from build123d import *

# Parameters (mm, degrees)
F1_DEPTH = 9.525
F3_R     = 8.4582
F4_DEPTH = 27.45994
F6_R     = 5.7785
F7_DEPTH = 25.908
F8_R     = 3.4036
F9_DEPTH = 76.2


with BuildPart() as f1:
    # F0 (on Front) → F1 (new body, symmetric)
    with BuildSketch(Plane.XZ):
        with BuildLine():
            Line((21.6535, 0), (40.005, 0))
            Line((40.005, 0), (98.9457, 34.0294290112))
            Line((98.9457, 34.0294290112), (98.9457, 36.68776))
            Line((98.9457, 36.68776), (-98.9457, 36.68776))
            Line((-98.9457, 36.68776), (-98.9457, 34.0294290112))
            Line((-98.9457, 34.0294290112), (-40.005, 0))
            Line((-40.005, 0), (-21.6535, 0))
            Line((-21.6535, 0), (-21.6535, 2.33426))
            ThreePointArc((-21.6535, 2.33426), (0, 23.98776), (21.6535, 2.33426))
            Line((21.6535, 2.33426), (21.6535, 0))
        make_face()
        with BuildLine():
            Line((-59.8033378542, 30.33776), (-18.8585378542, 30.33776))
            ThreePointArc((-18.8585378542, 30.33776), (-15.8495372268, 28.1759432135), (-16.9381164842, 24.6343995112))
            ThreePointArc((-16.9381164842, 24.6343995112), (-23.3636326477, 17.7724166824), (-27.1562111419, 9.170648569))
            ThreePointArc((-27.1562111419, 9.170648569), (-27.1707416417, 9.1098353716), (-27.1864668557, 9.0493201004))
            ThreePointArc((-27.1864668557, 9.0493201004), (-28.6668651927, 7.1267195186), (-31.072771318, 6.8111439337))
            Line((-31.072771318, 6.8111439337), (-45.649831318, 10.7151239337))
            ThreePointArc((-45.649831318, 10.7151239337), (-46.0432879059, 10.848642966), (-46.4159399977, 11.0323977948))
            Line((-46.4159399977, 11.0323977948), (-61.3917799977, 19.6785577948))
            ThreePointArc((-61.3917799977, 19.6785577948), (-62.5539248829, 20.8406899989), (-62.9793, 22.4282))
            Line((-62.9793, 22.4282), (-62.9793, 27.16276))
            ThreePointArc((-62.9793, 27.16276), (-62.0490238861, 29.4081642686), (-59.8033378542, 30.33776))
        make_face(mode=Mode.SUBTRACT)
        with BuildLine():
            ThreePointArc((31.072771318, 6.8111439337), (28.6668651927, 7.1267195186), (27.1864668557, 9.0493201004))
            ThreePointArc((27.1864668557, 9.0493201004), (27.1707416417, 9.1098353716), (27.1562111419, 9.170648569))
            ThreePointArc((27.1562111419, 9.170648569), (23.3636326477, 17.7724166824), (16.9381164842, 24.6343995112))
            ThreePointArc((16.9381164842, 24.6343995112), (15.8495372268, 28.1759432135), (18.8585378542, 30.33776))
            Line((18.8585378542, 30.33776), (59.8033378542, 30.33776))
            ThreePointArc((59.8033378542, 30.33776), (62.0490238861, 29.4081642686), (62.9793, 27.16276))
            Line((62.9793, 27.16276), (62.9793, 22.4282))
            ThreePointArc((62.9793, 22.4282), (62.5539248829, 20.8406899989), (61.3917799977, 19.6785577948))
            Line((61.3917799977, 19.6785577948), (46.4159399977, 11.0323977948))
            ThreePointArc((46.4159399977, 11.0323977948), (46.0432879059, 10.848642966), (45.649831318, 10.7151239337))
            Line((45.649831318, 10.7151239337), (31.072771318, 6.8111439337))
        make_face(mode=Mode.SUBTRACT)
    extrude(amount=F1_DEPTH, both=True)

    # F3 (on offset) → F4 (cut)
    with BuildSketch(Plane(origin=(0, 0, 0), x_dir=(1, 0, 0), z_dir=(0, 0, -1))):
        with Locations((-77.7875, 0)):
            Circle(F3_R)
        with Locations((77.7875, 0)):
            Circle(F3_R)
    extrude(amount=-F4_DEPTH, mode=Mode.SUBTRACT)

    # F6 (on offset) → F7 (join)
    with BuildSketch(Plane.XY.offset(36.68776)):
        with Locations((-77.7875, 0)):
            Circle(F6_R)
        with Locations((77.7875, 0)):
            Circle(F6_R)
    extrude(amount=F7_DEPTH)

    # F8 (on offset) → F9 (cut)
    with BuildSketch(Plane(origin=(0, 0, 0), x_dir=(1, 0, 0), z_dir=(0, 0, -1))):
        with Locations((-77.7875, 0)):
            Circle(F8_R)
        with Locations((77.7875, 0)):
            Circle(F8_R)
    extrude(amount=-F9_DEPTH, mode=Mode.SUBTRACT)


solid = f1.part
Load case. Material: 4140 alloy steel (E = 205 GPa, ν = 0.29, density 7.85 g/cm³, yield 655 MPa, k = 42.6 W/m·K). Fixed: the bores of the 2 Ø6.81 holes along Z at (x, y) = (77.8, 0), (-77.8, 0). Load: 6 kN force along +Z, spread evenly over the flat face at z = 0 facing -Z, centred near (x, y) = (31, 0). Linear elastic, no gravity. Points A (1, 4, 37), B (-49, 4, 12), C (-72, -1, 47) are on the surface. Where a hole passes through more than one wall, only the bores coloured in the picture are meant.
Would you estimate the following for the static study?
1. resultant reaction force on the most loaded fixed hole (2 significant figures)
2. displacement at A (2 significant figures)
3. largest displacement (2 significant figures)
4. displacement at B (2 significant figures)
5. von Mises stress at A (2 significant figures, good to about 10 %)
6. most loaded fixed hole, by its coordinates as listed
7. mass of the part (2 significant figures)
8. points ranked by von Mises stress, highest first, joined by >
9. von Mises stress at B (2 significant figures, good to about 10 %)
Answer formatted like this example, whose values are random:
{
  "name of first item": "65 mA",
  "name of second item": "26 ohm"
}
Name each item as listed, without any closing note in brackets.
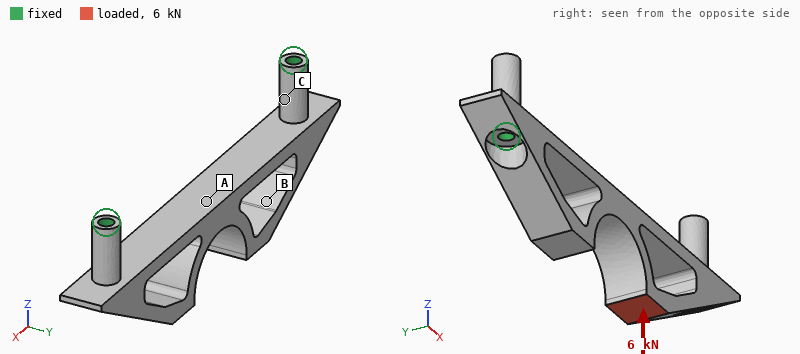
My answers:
{
  "resultant reaction force on the most loaded fixed hole": "4.5 kN",
  "displacement at A": "0.26 mm",
  "largest displacement": "0.27 mm",
  "displacement at B": "0.085 mm",
  "von Mises stress at A": "120 MPa",
  "most loaded fixed hole, by its coordinates as listed": "(77.8, 0)",
  "mass of the part": "430 g",
  "points ranked by von Mises stress, highest first, joined by >": "A > B > C",
  "von Mises stress at B": "64 MPa"
}
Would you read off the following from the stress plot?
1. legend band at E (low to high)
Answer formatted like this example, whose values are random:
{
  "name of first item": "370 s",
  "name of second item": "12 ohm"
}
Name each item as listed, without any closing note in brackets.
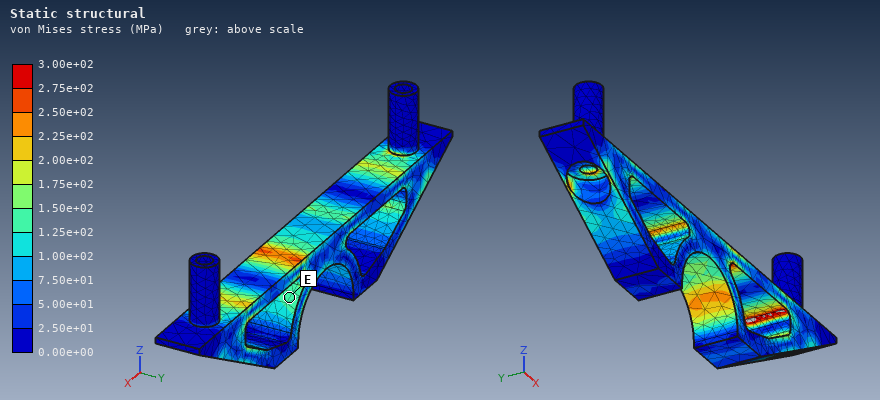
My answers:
{
  "legend band at E": "1.25e+02 to 1.50e+02 MPa"
}
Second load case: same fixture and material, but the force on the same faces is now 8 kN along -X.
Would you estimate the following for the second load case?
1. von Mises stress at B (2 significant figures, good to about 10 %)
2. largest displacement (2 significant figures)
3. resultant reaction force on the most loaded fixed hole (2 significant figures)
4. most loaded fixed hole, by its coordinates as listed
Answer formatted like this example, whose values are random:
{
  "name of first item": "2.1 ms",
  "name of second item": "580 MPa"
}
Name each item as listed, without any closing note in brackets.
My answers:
{
  "von Mises stress at B": "57 MPa",
  "largest displacement": "0.21 mm",
  "resultant reaction force on the most loaded fixed hole": "6.2 kN",
  "most loaded fixed hole, by its coordinates as listed": "(77.8, 0)"
}
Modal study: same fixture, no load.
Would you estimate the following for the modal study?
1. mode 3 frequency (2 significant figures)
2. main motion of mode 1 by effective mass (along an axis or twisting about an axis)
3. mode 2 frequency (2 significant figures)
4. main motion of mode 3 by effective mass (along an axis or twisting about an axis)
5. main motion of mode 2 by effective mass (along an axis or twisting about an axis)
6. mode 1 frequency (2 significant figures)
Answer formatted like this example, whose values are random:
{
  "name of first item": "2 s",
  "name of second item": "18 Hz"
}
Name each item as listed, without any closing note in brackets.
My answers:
{
  "mode 3 frequency": "4500 Hz",
  "main motion of mode 1 by effective mass": "along Z",
  "mode 2 frequency": "2600 Hz",
  "main motion of mode 3 by effective mass": "twisting about X",
  "main motion of mode 2 by effective mass": "along Y",
  "mode 1 frequency": "1600 Hz"
}
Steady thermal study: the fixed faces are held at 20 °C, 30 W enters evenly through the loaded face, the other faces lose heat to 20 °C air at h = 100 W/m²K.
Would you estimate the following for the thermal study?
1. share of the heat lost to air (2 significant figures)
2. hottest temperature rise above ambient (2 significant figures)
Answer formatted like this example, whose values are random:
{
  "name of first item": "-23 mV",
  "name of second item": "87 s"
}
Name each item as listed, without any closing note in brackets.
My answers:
{
  "share of the heat lost to air": "78 %",
  "hottest temperature rise above ambient": "80 K"
}
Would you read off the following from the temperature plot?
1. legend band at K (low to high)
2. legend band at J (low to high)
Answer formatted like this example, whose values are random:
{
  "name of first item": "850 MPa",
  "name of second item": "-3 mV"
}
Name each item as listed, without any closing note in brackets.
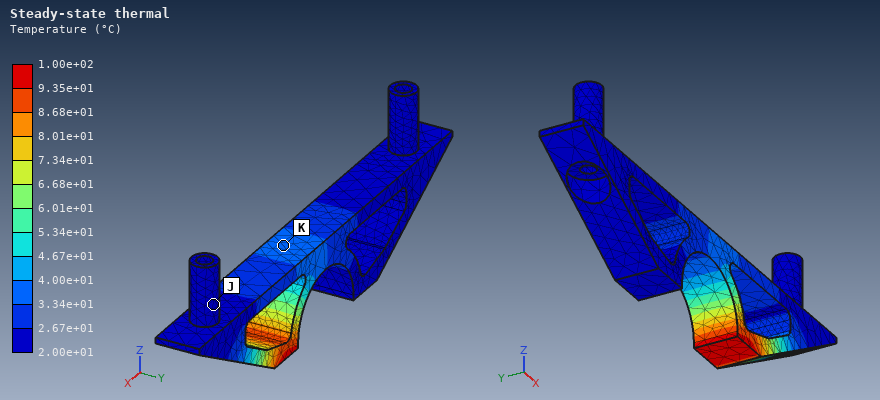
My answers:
{
  "legend band at K": "3.34e+01 to 4.00e+01 °C",
  "legend band at J": "2.00e+01 to 2.67e+01 °C"
}
